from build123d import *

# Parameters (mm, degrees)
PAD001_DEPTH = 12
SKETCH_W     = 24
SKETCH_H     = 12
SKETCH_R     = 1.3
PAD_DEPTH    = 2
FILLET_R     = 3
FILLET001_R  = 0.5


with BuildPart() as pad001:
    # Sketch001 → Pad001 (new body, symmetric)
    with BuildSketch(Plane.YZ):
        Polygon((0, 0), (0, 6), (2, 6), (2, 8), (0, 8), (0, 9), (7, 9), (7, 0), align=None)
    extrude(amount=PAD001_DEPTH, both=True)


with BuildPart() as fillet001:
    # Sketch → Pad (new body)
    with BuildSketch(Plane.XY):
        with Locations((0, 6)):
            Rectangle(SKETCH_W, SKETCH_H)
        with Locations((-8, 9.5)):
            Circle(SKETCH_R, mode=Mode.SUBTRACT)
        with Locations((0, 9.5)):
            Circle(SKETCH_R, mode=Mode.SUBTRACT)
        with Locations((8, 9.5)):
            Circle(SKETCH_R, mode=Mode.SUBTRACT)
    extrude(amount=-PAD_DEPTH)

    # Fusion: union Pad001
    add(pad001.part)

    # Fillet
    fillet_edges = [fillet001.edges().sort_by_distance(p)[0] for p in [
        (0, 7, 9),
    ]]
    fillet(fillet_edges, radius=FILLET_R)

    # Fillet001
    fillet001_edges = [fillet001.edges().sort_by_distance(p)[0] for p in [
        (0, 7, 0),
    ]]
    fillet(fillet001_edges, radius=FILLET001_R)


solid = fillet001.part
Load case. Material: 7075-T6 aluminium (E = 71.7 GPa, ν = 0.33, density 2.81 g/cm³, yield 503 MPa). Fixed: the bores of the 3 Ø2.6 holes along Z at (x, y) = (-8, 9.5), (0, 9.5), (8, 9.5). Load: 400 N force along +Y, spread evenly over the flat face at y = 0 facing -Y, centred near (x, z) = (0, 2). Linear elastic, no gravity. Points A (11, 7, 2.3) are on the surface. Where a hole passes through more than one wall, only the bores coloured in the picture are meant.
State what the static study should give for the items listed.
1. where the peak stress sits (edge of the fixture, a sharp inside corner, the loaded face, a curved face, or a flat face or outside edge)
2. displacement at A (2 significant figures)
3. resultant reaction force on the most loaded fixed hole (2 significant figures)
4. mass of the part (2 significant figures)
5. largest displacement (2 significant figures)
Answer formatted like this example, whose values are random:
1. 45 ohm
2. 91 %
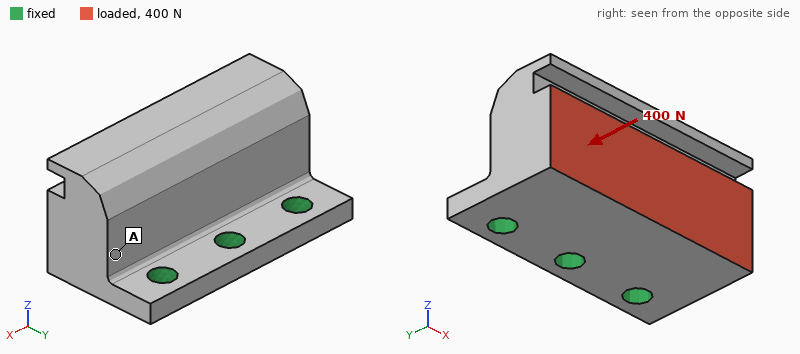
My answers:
1. a curved face
2. 9.2 µm
3. 130 N
4. 5.4 g
5. 34 µm
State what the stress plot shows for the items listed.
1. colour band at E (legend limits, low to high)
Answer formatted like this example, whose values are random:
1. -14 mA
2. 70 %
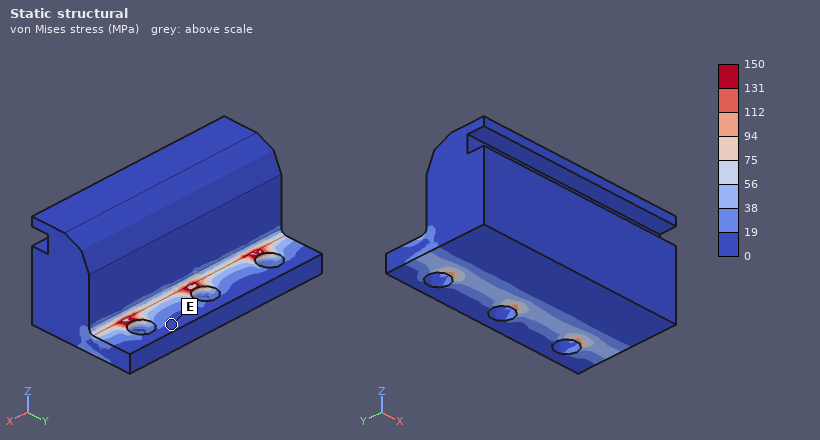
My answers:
1. 0 to 19 MPa
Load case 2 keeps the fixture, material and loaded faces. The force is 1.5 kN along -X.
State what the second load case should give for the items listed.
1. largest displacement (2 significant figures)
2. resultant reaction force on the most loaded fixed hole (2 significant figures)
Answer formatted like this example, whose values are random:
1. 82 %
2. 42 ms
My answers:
1. 15 µm
2. 920 N
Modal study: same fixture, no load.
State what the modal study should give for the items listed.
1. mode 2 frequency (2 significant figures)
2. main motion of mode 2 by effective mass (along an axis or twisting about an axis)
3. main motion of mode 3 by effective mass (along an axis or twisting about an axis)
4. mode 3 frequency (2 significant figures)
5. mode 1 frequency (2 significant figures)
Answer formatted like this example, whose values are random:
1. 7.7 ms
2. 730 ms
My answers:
1. 21 kHz
2. along X
3. along X
4. 31 kHz
5. 6900 Hz
